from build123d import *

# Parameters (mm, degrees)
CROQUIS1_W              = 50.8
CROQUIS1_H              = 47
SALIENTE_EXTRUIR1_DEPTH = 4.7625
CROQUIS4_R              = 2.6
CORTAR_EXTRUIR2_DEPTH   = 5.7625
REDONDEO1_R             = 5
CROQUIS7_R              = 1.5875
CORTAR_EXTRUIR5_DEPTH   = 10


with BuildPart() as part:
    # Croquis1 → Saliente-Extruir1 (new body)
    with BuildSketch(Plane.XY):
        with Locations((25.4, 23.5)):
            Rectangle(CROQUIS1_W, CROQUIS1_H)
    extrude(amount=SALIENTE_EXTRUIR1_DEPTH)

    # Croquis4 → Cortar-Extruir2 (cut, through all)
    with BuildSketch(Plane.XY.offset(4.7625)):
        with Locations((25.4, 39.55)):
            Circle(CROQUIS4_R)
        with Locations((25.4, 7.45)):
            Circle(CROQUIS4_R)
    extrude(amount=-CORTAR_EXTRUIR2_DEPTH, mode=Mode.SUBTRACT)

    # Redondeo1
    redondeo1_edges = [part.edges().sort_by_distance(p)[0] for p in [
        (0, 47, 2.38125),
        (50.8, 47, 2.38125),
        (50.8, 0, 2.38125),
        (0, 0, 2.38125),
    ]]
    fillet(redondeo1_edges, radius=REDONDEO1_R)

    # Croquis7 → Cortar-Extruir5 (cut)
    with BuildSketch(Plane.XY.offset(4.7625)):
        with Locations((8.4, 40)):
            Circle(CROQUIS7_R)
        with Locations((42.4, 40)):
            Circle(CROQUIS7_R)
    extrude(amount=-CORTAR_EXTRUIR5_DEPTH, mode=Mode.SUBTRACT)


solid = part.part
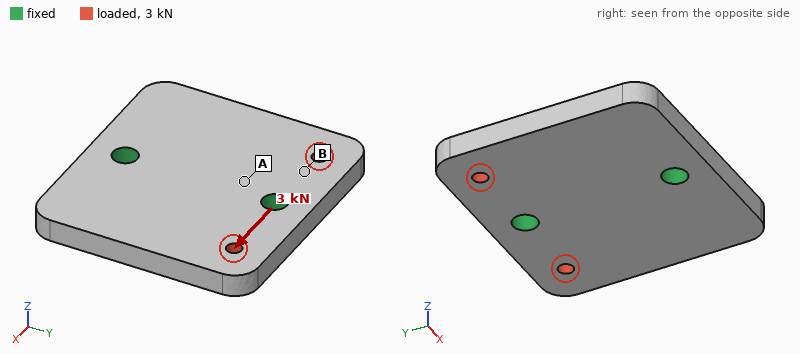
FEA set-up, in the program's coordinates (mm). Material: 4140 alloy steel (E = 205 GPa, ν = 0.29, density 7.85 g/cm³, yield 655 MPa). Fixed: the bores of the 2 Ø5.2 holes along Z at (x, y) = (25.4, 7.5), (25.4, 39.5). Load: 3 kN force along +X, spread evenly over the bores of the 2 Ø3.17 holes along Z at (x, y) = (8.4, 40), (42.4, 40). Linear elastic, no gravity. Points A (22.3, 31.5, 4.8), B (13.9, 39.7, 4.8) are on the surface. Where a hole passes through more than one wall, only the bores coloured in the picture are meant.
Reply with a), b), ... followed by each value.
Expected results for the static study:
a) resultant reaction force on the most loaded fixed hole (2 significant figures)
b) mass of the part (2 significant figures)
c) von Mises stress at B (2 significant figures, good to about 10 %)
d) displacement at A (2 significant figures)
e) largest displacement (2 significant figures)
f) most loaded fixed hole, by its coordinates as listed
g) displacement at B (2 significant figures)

a) 3.0 kN
b) 86 g
c) 30 MPa
d) 0.69 µm
e) 2.7 µm
f) (25.4, 39.5)
g) 1.5 µm
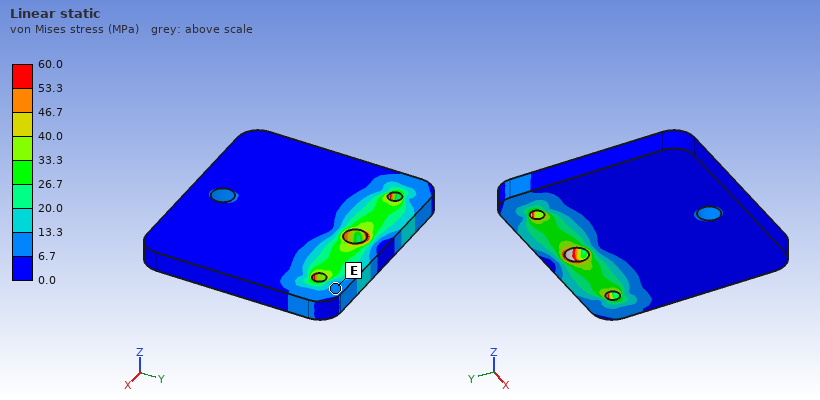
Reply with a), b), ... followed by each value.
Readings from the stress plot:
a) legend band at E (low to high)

a) 6.7 to 13.3 MPa
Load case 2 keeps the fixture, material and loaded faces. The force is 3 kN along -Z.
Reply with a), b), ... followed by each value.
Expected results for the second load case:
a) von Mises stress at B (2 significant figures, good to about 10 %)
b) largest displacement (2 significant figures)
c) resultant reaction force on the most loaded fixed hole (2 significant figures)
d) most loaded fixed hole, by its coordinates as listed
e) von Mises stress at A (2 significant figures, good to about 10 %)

a) 90 MPa
b) 74 µm
c) 3.0 kN
d) (25.4, 39.5)
e) 120 MPa
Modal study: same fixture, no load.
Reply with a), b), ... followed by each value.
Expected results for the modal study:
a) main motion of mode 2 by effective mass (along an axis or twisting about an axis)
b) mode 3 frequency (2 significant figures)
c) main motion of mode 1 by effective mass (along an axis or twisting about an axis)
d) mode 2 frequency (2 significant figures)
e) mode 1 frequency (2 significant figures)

a) along Z
b) 10 kHz
c) twisting about Y
d) 6500 Hz
e) 5500 Hz
